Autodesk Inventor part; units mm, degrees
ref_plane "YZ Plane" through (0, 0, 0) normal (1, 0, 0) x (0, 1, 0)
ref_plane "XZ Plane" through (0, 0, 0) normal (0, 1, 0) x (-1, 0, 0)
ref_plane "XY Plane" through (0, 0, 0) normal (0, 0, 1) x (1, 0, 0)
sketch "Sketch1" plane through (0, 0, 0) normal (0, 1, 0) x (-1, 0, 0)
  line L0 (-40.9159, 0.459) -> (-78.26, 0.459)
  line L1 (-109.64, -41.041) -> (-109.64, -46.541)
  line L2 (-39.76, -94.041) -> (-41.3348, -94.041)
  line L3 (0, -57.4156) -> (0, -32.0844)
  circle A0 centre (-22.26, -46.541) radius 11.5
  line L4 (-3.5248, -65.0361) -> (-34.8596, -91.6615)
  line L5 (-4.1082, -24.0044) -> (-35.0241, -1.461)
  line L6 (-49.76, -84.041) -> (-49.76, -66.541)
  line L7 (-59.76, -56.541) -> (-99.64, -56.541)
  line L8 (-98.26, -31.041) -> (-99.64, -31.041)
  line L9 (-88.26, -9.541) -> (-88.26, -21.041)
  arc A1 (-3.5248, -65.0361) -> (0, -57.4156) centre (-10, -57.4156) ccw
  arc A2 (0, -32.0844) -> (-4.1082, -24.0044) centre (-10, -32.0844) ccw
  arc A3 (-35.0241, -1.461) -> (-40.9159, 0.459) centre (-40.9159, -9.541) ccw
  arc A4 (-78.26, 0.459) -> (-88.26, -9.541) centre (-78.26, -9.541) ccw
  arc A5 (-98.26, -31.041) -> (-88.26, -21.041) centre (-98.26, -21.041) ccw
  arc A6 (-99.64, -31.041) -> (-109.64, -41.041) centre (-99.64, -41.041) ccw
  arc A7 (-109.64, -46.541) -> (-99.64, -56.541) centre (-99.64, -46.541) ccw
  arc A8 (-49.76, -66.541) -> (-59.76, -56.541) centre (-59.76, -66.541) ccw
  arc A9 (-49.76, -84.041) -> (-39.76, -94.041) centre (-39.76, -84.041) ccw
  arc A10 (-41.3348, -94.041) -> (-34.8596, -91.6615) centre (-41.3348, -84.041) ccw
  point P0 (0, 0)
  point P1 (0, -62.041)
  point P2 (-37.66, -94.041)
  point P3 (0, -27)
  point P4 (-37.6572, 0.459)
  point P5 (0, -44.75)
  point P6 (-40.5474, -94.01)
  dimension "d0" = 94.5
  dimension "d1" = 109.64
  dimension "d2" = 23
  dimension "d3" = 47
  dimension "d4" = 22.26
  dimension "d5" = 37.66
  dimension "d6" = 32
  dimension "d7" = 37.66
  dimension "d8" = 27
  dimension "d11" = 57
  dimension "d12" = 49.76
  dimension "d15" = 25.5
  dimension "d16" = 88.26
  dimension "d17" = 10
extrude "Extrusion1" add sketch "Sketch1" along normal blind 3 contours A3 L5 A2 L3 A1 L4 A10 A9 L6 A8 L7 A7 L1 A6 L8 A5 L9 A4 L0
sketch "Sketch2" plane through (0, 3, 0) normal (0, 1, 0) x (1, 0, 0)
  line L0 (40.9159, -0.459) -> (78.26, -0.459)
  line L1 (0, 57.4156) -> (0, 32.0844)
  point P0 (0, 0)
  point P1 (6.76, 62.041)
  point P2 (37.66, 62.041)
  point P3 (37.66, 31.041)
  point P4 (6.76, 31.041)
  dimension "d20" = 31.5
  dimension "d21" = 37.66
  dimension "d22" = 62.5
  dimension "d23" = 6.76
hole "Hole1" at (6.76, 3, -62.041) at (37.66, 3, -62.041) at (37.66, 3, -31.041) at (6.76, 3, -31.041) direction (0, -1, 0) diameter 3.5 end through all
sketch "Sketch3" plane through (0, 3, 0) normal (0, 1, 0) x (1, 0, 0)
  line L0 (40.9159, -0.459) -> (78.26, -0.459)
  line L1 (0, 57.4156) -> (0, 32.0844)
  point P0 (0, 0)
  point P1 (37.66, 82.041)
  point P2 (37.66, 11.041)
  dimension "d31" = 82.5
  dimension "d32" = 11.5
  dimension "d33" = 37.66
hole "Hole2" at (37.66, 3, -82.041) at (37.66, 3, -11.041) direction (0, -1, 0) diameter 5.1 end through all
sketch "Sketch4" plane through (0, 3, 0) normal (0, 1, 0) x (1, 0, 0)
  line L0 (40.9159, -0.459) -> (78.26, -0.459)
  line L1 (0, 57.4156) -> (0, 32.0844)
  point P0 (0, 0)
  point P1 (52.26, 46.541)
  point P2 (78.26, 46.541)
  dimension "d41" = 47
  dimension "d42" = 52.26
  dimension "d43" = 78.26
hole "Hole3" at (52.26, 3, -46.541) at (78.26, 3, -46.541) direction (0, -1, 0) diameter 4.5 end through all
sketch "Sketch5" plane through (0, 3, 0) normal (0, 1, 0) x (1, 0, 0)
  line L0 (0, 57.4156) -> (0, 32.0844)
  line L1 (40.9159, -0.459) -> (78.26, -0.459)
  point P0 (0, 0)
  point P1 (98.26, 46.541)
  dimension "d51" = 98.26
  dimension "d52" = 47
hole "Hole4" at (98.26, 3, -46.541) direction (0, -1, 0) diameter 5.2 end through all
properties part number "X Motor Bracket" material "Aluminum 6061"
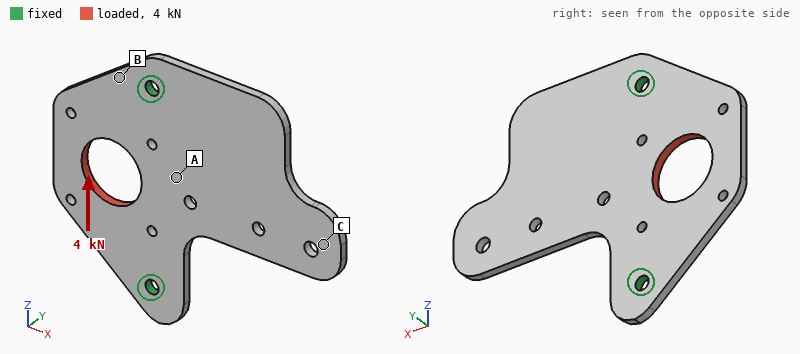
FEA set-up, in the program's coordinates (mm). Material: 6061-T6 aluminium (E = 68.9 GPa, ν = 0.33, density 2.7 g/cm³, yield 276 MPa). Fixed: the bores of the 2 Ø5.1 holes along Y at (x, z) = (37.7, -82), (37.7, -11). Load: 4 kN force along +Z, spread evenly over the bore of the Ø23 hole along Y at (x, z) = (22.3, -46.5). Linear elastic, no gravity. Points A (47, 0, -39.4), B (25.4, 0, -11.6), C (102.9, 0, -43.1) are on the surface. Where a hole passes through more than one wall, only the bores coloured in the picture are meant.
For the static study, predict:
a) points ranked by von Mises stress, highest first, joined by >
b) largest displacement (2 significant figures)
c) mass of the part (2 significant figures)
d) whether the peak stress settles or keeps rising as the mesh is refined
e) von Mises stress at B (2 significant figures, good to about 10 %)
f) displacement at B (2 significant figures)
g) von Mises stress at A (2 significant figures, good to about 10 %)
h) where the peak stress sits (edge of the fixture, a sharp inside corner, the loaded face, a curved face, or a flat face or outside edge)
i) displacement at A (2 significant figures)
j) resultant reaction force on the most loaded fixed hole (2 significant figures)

B > A > C
33 µm
46 g
keeps rising
28 MPa
11 µm
12 MPa
edge of the fixture
6.7 µm
2.2 kN
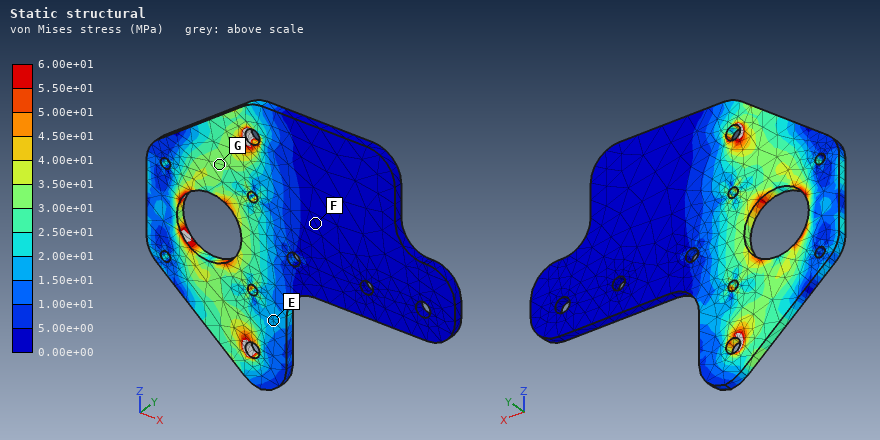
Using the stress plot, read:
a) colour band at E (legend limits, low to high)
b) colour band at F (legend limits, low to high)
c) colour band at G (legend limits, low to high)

1.50e+01 to 2.00e+01 MPa
0.00e+00 to 5.00e+00 MPa
3.00e+01 to 3.50e+01 MPa
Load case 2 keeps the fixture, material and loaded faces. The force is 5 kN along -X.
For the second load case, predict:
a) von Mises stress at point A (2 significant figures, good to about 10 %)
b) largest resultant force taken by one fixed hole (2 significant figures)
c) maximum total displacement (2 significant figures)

28 MPa
2.6 kN
63 µm
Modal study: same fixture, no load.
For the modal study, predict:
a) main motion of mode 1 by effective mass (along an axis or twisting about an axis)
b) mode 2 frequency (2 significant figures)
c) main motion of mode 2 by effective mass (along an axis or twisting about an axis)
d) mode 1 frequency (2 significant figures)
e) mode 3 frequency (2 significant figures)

along Y
1600 Hz
along Y
560 Hz
1900 Hz
